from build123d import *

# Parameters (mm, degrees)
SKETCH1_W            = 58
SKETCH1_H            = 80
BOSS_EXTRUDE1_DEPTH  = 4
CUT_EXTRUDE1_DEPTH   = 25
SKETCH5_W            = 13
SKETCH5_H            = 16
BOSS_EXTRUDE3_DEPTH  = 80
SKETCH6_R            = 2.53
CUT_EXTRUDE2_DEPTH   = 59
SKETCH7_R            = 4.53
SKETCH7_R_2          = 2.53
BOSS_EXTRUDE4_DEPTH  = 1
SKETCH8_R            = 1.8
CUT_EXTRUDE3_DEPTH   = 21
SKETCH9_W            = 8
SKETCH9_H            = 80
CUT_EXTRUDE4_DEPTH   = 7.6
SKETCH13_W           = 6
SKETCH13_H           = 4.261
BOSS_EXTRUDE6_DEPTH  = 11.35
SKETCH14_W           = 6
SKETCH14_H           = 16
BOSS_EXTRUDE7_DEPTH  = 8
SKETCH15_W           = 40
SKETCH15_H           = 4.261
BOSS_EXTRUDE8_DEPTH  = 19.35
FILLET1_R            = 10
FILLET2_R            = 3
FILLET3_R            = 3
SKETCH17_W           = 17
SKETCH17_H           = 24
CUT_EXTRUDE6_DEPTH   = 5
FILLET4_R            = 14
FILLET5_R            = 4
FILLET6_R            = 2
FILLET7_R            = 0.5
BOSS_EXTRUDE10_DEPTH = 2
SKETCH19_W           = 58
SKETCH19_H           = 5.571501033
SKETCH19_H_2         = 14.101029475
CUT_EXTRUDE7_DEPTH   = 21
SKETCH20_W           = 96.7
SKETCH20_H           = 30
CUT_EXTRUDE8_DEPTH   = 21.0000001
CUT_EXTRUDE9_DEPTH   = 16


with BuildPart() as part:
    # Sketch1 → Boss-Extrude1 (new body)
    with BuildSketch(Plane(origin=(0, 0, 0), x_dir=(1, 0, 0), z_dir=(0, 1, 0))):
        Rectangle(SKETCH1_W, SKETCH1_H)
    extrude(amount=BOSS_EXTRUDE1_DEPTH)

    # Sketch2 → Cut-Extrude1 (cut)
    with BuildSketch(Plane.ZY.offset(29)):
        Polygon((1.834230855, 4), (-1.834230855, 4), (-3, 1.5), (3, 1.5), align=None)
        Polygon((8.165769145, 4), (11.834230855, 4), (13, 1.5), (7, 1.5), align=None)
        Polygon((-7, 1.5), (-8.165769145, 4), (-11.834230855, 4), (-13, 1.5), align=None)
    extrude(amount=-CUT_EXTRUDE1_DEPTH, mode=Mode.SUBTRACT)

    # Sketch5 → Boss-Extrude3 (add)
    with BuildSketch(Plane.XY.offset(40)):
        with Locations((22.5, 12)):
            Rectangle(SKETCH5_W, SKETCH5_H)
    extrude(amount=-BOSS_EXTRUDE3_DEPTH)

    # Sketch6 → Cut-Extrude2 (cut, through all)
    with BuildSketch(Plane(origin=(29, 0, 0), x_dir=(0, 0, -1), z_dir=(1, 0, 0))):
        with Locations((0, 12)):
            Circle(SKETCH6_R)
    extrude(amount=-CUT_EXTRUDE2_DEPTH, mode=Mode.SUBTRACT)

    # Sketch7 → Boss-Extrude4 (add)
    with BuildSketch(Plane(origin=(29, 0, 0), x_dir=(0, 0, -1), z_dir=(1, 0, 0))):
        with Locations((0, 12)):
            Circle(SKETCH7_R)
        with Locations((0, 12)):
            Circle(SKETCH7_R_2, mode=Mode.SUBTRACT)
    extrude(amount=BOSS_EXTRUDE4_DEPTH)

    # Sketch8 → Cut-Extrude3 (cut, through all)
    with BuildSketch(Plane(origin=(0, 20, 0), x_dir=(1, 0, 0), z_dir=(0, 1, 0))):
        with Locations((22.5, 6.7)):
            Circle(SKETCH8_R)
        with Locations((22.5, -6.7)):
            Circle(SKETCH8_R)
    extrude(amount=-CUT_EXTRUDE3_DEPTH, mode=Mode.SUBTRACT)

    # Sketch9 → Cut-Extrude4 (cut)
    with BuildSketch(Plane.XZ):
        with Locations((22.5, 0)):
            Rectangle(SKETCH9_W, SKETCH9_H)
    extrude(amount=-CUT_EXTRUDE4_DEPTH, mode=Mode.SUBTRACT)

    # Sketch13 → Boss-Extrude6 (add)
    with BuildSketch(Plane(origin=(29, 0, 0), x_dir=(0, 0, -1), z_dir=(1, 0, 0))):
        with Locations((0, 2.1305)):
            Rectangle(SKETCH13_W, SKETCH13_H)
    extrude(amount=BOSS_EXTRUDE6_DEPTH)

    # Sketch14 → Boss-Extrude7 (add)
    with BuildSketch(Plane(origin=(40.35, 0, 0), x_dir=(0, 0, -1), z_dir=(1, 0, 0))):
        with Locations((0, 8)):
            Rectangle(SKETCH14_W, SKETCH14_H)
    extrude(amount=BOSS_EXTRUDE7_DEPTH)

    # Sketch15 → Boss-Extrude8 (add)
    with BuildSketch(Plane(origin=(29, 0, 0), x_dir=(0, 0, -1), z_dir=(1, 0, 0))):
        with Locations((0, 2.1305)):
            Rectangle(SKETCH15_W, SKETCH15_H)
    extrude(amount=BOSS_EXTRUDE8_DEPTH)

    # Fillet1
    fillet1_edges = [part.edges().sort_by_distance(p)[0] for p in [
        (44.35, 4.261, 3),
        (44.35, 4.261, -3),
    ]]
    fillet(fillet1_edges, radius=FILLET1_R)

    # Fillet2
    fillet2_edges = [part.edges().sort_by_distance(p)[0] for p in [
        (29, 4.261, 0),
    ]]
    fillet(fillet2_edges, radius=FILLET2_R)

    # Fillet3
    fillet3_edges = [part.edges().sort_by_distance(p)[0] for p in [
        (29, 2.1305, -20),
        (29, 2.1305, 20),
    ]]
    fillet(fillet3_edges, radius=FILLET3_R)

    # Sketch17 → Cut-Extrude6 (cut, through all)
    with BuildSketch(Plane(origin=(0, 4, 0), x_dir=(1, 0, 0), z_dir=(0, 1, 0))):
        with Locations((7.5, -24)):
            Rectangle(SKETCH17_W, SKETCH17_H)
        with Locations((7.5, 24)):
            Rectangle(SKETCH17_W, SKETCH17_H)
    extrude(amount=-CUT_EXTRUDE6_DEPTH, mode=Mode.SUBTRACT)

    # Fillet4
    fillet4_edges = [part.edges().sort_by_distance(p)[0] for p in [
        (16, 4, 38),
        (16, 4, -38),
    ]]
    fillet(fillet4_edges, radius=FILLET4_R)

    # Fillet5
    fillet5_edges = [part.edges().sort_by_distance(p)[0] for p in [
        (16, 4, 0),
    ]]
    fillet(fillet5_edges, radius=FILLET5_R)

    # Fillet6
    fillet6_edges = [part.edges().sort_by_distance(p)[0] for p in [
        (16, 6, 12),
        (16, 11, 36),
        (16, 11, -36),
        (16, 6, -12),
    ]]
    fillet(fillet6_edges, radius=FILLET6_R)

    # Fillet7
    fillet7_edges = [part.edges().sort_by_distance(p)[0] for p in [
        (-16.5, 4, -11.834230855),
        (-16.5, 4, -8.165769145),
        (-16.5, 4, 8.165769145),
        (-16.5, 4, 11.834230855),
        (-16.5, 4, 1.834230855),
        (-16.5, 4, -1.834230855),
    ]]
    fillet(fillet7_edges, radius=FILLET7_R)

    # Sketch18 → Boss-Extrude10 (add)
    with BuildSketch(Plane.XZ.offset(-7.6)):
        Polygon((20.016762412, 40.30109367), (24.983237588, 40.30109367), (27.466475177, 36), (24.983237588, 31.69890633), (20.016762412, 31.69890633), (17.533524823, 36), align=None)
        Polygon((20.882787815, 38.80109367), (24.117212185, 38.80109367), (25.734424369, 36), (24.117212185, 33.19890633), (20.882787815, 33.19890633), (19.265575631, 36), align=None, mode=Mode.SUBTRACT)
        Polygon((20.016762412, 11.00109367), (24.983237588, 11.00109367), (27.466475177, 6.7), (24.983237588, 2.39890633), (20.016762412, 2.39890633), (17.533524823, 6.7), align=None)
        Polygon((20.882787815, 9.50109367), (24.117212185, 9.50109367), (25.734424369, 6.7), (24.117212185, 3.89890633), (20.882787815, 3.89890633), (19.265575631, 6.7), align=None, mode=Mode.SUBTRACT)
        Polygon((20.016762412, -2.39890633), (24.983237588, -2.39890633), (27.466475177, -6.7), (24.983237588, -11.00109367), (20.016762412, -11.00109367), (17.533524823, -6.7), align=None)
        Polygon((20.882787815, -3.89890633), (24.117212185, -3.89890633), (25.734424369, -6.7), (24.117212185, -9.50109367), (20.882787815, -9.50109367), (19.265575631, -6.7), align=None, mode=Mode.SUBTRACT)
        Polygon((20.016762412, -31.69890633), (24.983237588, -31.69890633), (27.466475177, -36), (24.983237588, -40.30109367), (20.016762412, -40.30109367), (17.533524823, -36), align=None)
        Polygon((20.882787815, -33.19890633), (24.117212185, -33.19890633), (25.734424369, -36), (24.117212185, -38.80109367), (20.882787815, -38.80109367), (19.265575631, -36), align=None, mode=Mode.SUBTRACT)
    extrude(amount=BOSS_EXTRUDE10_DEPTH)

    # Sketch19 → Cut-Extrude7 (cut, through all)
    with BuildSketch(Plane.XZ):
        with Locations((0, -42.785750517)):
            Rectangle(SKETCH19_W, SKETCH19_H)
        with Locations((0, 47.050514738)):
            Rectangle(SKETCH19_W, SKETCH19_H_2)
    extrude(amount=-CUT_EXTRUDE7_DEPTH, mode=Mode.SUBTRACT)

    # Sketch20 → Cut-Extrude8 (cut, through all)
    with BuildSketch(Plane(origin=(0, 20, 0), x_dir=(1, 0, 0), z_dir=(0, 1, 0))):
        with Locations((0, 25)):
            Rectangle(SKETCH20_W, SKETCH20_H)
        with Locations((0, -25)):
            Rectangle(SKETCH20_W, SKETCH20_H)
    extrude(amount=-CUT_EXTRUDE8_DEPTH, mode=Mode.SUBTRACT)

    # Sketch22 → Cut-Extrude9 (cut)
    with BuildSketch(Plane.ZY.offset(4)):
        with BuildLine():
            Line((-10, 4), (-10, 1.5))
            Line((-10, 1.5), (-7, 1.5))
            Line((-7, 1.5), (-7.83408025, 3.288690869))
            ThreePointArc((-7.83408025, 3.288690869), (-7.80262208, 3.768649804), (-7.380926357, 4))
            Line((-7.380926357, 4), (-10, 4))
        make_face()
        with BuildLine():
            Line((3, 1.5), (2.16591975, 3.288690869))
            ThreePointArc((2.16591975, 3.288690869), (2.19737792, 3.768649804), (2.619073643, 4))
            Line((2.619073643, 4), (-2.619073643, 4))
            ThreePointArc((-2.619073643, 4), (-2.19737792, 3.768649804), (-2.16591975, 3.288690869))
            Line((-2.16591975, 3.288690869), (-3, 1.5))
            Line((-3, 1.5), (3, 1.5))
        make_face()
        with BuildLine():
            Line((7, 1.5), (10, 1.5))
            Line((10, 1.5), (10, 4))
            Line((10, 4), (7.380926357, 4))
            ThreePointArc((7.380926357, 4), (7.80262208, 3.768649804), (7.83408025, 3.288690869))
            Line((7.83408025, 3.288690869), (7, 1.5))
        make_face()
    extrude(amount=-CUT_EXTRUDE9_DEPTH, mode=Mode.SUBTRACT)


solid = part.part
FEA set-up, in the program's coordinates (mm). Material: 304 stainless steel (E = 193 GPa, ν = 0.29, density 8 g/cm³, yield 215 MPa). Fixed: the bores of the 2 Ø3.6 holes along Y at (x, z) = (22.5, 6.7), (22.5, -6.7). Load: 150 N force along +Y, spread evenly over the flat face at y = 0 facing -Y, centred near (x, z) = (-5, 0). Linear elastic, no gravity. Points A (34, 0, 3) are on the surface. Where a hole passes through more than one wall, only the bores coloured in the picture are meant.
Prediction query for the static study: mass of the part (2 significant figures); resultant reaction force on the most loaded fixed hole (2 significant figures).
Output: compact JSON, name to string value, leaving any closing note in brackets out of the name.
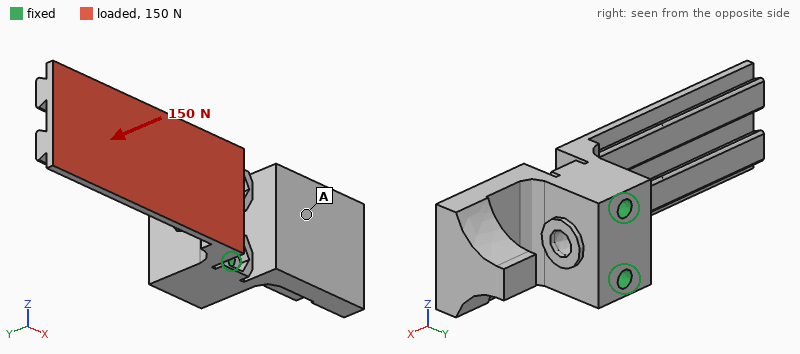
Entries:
{"mass of the part": "71 g", "resultant reaction force on the most loaded fixed hole": "80 N"}
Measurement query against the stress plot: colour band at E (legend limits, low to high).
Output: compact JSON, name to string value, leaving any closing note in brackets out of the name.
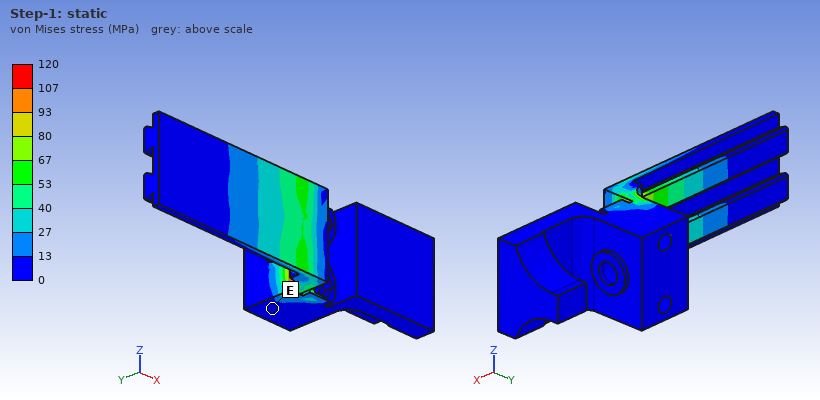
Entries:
{"colour band at E": "0 to 13 MPa"}
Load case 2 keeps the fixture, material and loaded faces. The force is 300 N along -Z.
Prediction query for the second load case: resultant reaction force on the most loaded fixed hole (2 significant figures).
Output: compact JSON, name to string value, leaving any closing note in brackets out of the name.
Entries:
{"resultant reaction force on the most loaded fixed hole": "600 N"}
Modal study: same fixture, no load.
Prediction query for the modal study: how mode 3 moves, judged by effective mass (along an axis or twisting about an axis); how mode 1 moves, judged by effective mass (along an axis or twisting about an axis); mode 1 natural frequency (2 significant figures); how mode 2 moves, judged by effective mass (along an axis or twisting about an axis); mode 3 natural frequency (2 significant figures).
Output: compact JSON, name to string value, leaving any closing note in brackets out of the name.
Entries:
{"how mode 3 moves, judged by effective mass": "along Z", "how mode 1 moves, judged by effective mass": "along Y", "mode 1 natural frequency": "1200 Hz", "how mode 2 moves, judged by effective mass": "along Y", "mode 3 natural frequency": "3300 Hz"}
